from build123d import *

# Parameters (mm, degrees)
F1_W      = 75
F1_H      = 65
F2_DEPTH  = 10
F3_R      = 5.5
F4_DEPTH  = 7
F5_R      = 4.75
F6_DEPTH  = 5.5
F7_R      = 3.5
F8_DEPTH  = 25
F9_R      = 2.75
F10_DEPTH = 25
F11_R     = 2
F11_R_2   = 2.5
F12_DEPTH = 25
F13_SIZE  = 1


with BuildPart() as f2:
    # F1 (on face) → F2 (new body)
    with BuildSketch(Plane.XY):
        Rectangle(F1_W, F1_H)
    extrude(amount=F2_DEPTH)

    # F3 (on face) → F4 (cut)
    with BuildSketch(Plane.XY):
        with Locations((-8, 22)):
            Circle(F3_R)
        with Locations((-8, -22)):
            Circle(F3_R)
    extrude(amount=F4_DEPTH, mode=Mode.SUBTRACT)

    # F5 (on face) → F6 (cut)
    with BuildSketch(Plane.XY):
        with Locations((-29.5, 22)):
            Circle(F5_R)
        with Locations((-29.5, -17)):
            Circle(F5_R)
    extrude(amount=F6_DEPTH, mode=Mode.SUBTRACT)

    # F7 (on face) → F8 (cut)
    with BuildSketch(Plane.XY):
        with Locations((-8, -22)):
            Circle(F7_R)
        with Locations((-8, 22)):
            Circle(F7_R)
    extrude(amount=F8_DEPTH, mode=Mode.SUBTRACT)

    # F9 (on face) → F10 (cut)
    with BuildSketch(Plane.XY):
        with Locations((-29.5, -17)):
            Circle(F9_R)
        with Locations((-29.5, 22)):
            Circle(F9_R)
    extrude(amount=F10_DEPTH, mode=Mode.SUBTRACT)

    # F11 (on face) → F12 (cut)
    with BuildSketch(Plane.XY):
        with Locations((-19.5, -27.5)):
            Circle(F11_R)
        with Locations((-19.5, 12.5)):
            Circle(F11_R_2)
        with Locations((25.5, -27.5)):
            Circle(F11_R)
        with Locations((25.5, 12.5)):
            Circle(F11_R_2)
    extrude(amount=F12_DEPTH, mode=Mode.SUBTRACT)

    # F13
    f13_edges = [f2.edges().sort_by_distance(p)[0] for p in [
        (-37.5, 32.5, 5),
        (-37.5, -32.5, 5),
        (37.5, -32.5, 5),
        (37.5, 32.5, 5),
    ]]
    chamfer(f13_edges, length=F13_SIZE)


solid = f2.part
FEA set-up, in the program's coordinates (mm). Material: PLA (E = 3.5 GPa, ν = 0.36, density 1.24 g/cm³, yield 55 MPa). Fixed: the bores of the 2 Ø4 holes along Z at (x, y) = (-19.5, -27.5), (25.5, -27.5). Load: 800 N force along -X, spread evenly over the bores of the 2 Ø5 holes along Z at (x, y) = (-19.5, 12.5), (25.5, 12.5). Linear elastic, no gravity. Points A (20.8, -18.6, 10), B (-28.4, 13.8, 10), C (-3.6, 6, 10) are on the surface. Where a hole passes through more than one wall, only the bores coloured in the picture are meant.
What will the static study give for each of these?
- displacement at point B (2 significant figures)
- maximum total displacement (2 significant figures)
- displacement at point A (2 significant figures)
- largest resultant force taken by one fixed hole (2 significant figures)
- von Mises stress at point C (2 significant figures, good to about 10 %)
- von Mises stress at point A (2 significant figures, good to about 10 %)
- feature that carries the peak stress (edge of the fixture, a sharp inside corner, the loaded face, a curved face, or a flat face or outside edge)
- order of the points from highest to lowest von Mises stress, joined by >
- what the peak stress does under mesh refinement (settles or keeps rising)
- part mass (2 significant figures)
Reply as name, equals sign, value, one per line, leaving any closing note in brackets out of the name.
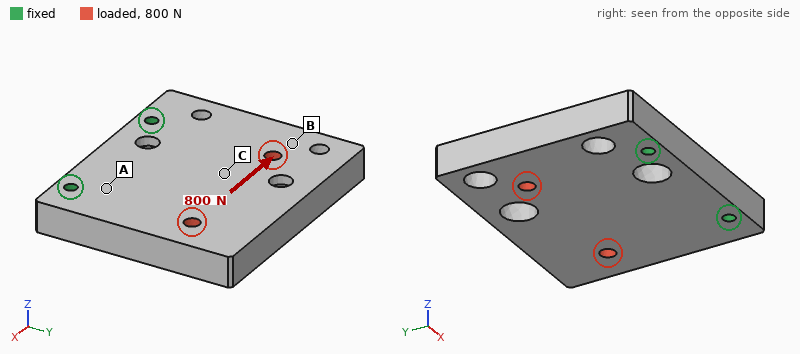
displacement at point B = 0.10 mm
maximum total displacement = 0.13 mm
displacement at point A = 0.022 mm
largest resultant force taken by one fixed hole = 810 N
von Mises stress at point C = 2.8 MPa
von Mises stress at point A = 4.7 MPa
feature that carries the peak stress = edge of the fixture
order of the points from highest to lowest von Mises stress, joined by > = A > C > B
what the peak stress does under mesh refinement = keeps rising
part mass = 56 g
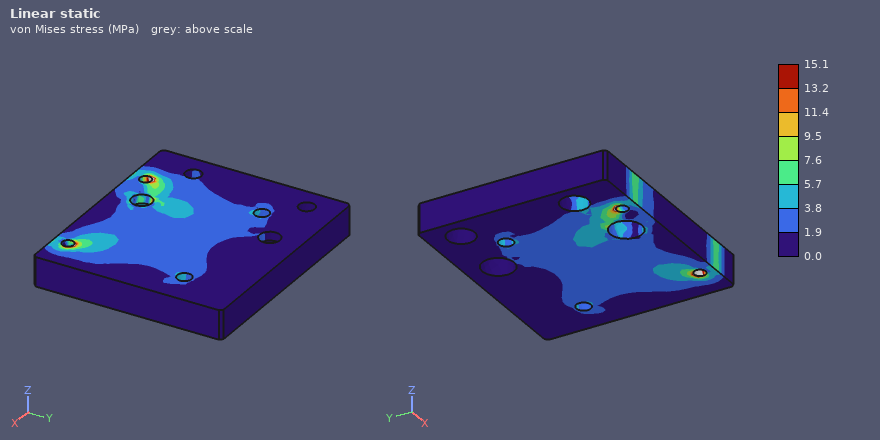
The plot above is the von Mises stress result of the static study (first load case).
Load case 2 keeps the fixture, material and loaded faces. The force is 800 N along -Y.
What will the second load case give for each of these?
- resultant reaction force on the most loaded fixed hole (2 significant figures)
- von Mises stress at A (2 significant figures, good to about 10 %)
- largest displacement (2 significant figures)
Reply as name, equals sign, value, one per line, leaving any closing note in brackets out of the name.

resultant reaction force on the most loaded fixed hole = 400 N
von Mises stress at A = 2.0 MPa
largest displacement = 30 µm
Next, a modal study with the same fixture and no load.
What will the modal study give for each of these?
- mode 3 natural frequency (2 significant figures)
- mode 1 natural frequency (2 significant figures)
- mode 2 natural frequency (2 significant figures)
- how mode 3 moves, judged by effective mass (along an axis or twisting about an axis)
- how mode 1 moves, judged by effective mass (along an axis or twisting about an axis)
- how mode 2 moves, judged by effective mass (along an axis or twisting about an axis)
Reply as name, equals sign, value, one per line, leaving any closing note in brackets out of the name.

mode 3 natural frequency = 2300 Hz
mode 1 natural frequency = 590 Hz
mode 2 natural frequency = 1300 Hz
how mode 3 moves, judged by effective mass = along X
how mode 1 moves, judged by effective mass = along Z
how mode 2 moves, judged by effective mass = twisting about Y
